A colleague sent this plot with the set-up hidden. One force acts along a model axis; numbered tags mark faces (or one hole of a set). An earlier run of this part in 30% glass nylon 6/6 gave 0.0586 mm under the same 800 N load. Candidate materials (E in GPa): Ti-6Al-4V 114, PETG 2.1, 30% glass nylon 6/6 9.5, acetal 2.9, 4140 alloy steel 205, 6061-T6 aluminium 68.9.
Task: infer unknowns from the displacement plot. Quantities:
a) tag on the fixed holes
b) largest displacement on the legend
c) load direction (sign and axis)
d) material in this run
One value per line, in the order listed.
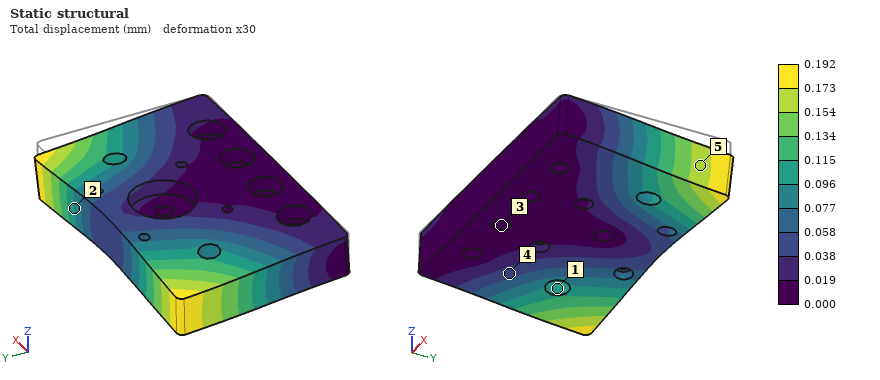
3
0.192 mm
-Z
acetal
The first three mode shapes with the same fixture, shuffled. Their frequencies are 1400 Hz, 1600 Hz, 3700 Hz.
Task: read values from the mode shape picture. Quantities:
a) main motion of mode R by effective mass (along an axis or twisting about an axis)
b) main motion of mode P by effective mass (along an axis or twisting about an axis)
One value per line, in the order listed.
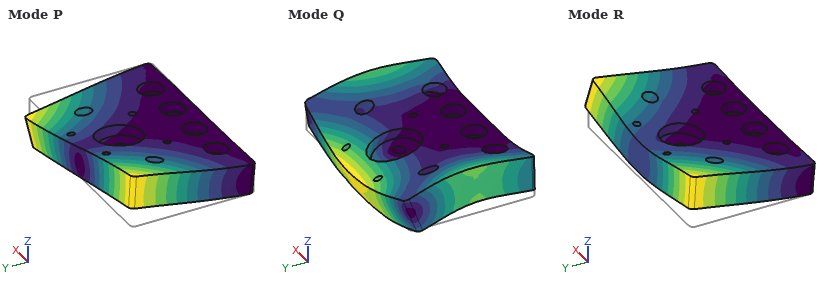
along Z
twisting about Y
